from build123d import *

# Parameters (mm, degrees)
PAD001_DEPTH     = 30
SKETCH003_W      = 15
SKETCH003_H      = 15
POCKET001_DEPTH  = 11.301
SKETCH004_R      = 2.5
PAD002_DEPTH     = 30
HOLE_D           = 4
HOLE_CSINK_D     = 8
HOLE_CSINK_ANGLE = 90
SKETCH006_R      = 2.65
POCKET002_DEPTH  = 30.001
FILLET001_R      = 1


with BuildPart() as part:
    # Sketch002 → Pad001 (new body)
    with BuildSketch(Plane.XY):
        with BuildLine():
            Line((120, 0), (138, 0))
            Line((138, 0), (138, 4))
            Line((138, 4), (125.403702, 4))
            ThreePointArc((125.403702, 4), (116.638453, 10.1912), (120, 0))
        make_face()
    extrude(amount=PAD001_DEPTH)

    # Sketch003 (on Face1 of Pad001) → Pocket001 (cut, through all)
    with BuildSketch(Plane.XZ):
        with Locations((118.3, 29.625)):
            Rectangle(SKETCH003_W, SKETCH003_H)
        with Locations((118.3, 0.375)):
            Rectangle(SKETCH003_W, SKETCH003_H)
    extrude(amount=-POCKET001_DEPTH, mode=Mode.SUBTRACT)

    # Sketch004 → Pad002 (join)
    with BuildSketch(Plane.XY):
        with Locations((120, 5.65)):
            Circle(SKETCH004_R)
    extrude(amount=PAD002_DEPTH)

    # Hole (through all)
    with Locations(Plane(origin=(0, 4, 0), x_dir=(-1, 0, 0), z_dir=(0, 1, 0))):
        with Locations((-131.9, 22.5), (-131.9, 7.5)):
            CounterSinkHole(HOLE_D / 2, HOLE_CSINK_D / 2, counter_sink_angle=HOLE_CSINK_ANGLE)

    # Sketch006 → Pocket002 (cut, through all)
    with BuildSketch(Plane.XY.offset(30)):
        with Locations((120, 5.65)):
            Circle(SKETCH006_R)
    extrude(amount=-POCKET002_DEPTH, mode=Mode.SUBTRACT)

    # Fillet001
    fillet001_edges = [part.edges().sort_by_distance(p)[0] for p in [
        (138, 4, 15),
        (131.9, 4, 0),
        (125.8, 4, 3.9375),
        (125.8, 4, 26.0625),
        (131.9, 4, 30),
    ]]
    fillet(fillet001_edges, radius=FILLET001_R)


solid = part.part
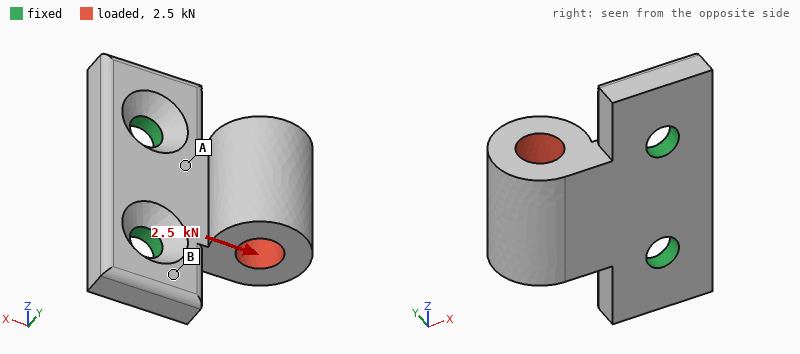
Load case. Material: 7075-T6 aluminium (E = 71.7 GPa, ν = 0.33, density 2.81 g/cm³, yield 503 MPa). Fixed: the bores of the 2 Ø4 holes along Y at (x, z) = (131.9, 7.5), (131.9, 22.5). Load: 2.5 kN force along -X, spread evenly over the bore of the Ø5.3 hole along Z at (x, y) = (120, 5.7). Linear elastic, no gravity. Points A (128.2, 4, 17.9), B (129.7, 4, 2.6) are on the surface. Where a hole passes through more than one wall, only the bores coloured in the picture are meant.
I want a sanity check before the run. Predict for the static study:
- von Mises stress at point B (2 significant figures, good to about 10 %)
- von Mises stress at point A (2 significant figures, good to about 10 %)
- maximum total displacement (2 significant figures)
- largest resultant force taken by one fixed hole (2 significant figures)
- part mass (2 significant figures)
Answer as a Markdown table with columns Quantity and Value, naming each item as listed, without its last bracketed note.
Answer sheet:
| Quantity | Value |
|---|---|
| von Mises stress at point B | 63 MPa |
| von Mises stress at point A | 230 MPa |
| maximum total displacement | 0.26 mm |
| largest resultant force taken by one fixed hole | 1.3 kN |
| part mass | 7.0 g |
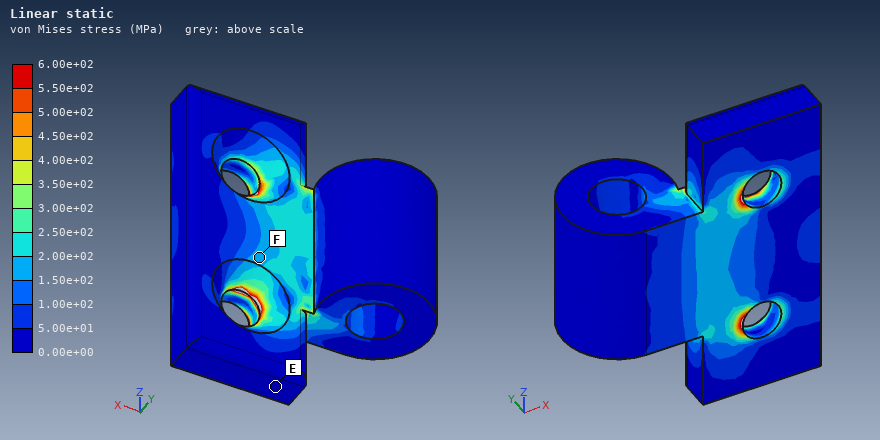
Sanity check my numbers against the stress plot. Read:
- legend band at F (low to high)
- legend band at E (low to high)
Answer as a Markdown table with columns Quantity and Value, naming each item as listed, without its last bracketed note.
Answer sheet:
| Quantity | Value |
|---|---|
| legend band at F | 1.50e+02 to 2.00e+02 MPa |
| legend band at E | 0.00e+00 to 5.00e+01 MPa |
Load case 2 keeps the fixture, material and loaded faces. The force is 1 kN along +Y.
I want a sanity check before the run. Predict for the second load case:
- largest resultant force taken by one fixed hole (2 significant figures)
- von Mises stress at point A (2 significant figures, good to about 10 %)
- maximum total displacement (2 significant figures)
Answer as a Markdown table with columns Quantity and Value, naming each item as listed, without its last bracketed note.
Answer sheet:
| Quantity | Value |
|---|---|
| largest resultant force taken by one fixed hole | 560 N |
| von Mises stress at point A | 180 MPa |
| maximum total displacement | 0.22 mm |
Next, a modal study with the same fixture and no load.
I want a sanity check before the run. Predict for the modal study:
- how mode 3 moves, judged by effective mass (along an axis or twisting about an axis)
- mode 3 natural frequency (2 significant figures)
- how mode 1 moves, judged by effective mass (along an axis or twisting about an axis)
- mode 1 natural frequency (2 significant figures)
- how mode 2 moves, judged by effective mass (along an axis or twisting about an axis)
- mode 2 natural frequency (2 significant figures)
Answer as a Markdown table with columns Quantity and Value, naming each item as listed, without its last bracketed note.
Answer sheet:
| Quantity | Value |
|---|---|
| how mode 3 moves, judged by effective mass | along Z |
| mode 3 natural frequency | 29 kHz |
| how mode 1 moves, judged by effective mass | along Y |
| mode 1 natural frequency | 6500 Hz |
| how mode 2 moves, judged by effective mass | along Z |
| mode 2 natural frequency | 20 kHz |
